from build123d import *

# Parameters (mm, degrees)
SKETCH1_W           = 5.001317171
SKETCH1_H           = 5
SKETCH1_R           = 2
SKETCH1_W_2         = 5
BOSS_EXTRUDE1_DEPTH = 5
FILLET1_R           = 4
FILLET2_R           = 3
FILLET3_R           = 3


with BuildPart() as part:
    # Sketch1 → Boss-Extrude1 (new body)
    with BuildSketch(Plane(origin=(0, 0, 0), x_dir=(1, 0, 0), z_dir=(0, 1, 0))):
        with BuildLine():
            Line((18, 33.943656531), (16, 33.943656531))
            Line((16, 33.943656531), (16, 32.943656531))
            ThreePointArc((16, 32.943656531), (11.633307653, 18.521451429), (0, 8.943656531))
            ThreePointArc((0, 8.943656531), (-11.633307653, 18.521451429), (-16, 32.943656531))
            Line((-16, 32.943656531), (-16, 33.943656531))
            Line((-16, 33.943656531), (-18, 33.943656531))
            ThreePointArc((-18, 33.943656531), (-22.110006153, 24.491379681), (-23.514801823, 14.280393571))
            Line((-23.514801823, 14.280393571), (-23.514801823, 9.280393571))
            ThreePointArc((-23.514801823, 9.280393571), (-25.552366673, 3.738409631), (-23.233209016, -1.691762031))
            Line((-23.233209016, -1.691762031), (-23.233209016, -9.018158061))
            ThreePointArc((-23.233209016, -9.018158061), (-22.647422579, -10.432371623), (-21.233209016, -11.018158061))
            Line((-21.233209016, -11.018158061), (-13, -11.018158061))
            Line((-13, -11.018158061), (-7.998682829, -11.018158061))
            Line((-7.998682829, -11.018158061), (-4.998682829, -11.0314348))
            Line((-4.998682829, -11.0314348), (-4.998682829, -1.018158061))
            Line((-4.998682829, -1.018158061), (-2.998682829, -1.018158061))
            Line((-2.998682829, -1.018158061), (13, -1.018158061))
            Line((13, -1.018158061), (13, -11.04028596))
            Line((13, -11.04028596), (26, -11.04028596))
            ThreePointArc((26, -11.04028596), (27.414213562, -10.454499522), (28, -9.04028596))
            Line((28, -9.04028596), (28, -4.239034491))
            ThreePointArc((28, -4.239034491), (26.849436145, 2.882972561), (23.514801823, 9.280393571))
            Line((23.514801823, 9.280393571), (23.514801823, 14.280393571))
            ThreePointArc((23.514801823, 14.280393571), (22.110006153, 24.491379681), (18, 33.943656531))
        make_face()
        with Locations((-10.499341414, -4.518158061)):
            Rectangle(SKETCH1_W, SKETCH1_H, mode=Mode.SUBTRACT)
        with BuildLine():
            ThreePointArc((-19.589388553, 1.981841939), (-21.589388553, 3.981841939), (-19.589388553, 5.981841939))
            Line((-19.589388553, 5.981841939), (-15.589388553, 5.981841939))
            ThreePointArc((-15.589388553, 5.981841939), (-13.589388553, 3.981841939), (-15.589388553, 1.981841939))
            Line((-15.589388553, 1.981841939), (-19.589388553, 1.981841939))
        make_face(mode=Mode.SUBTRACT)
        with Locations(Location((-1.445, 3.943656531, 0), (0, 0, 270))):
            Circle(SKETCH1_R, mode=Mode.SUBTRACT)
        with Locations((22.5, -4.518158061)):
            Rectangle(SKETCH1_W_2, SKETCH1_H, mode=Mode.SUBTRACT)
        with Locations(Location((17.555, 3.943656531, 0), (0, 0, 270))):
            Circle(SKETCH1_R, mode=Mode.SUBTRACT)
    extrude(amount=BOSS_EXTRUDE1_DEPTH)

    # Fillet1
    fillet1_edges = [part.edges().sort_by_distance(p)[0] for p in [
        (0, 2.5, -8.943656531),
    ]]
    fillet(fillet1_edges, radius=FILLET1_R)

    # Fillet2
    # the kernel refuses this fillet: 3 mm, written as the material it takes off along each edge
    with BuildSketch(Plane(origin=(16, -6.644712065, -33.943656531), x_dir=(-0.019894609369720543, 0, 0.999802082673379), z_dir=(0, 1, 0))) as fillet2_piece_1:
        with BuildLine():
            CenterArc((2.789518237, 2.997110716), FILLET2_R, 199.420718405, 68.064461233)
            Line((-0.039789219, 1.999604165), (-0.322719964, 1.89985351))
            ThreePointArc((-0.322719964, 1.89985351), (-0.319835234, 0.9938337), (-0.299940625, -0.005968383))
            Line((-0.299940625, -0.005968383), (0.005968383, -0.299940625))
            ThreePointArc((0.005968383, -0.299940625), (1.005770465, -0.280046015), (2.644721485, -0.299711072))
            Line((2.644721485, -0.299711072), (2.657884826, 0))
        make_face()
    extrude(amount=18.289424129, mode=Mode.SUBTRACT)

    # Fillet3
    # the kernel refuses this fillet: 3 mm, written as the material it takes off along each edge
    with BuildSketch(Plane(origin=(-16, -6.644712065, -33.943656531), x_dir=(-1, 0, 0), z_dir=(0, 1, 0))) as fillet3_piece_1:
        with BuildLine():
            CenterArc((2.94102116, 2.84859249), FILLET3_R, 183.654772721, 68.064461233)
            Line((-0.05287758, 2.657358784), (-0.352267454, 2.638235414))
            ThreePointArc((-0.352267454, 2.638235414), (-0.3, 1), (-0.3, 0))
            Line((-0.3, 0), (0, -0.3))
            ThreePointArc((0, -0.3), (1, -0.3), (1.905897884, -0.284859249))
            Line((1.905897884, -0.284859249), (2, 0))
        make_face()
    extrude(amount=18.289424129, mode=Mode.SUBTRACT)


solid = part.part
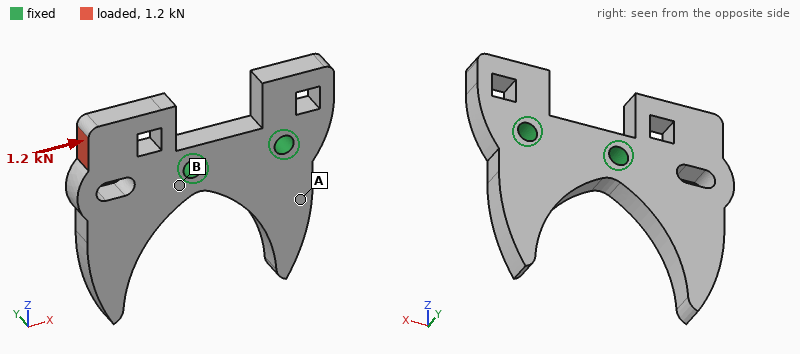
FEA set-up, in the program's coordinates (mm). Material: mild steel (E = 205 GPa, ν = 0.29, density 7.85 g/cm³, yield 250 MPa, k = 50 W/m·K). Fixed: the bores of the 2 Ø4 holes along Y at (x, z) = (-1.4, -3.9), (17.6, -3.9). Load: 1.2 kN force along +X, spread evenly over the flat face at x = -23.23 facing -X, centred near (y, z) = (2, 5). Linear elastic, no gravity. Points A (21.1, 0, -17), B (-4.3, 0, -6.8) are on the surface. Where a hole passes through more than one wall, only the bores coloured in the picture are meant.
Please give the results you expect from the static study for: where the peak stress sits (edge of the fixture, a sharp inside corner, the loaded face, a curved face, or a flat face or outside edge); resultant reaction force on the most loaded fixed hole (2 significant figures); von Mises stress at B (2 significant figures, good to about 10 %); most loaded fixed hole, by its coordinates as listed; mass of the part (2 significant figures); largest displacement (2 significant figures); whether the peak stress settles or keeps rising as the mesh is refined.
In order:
edge of the fixture
1.3 kN
37 MPa
(-1.4, -3.9)
49 g
33 µm
keeps rising
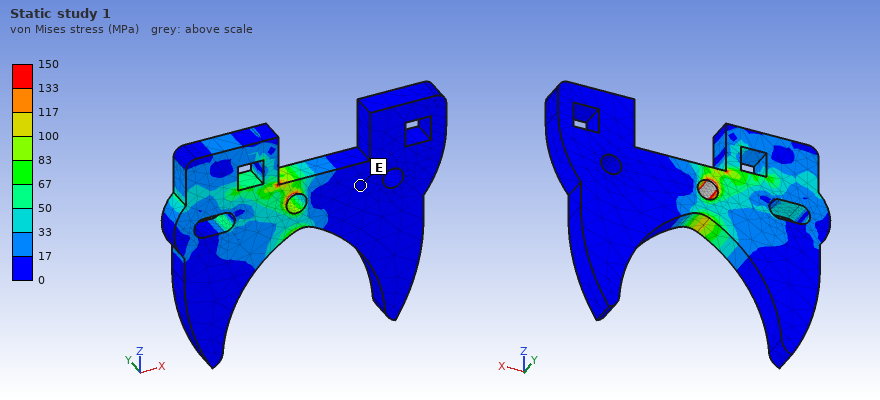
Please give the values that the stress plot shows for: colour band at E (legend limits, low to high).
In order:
0 to 17 MPa
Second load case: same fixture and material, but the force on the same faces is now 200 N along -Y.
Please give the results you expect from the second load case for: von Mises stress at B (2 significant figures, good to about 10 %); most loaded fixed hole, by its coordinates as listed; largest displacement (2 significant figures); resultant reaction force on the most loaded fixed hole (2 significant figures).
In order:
60 MPa
(-1.4, -3.9)
37 µm
220 N
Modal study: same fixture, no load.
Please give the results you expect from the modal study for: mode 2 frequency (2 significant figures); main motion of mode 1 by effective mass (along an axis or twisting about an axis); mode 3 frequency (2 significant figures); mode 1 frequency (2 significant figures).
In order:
6200 Hz
along Y
6400 Hz
4300 Hz
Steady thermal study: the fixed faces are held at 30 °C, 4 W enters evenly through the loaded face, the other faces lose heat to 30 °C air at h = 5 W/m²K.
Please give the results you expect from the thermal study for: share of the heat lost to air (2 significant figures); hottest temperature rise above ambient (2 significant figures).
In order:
3.2 %
31 K
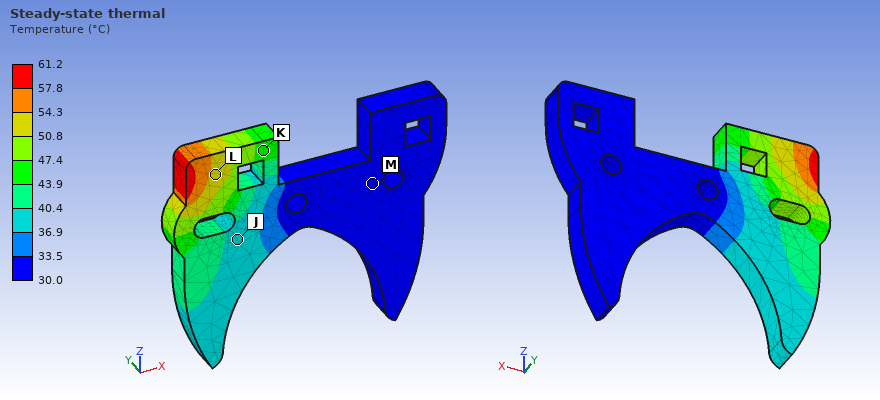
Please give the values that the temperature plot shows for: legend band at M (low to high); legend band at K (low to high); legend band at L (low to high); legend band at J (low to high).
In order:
30.0 to 33.5 °C
43.9 to 47.4 °C
50.8 to 54.3 °C
36.9 to 40.4 °C
